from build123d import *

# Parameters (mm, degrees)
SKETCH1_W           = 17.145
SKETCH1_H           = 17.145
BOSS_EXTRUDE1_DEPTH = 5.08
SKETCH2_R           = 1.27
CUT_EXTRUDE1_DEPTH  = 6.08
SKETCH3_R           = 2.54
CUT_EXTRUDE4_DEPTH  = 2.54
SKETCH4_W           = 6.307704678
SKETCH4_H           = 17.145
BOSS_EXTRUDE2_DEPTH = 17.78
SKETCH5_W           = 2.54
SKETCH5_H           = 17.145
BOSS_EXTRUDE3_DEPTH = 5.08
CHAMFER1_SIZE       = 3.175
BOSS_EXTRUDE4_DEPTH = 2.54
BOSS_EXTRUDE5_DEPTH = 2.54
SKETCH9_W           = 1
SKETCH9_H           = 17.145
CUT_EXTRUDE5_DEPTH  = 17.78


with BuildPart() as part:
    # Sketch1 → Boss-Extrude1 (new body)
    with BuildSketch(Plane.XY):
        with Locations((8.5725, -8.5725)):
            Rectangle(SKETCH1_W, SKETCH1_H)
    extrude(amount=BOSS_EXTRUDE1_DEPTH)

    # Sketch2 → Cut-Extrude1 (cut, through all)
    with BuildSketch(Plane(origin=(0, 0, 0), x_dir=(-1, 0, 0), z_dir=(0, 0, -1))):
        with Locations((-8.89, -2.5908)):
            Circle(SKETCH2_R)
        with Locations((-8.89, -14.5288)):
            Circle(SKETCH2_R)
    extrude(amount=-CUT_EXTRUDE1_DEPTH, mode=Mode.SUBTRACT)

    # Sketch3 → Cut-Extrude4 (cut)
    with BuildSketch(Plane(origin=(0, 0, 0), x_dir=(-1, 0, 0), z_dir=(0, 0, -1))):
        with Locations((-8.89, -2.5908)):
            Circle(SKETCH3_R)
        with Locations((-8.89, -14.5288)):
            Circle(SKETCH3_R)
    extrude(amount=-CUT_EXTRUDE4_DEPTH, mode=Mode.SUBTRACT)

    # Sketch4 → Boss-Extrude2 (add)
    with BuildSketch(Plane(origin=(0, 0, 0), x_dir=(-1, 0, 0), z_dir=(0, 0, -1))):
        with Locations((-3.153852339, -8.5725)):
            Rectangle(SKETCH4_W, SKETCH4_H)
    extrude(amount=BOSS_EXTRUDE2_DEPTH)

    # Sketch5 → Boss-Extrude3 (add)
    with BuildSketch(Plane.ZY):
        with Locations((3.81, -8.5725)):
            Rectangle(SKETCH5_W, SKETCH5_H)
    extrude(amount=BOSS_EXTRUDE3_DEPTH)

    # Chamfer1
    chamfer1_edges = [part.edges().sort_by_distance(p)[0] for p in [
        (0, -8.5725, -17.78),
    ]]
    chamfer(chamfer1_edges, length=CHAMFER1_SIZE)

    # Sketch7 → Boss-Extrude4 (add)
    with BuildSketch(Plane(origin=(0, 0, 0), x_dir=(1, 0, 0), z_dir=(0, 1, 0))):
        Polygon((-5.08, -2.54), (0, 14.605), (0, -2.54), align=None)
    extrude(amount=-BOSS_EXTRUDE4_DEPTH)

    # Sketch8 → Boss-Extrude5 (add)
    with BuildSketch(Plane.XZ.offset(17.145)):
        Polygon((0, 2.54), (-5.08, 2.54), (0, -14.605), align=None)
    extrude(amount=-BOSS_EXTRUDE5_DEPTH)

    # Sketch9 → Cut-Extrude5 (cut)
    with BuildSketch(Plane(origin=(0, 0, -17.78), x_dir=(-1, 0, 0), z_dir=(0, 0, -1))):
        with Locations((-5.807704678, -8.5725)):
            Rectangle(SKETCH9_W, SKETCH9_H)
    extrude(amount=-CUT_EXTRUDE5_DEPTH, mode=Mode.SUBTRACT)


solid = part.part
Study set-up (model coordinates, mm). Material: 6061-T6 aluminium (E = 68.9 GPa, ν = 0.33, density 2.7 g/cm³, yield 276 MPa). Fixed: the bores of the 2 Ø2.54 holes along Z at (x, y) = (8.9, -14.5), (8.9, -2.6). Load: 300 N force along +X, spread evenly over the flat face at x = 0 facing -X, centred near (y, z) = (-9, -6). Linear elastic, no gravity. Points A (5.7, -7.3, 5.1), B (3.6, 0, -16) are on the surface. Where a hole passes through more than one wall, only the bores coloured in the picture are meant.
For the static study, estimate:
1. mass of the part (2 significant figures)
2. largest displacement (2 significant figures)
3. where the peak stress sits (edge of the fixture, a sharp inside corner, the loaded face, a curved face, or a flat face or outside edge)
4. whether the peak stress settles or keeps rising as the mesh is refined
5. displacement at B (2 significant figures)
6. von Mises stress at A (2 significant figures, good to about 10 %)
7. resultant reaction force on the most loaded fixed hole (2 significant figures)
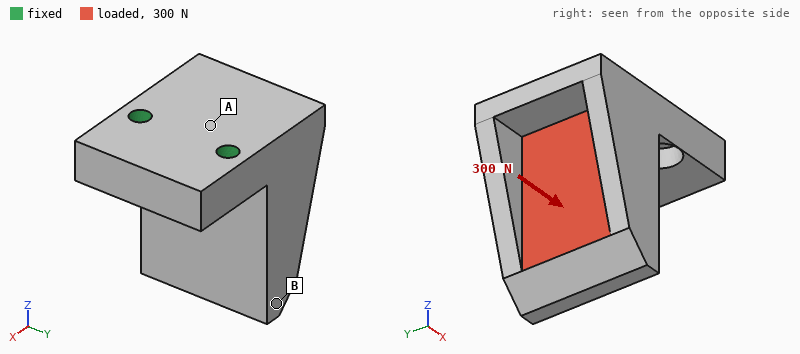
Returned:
9.0 g
73 µm
edge of the fixture
keeps rising
66 µm
34 MPa
150 N
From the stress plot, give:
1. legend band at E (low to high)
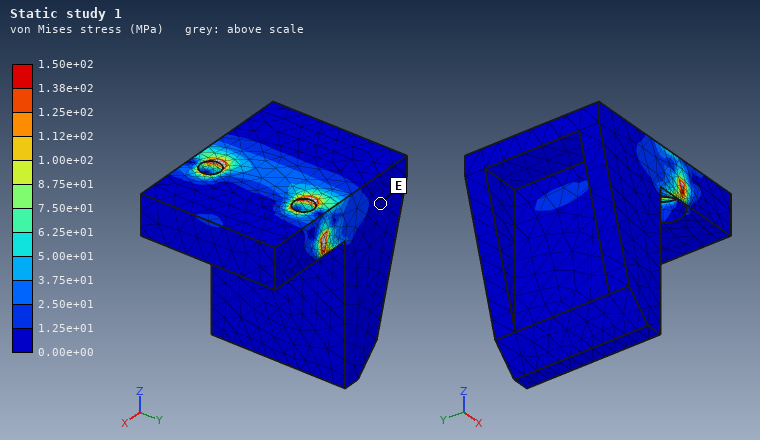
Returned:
0.00e+00 to 1.25e+01 MPa
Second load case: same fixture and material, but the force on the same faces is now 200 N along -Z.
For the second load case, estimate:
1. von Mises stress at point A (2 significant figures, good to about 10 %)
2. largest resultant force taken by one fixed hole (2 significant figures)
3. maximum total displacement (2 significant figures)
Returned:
16 MPa
100 N
36 µm
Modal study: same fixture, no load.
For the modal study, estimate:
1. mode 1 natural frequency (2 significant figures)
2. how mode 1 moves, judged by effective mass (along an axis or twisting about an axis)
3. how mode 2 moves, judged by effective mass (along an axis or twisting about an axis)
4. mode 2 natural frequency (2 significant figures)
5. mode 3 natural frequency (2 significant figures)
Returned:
4800 Hz
along X
along Y
11 kHz
21 kHz
